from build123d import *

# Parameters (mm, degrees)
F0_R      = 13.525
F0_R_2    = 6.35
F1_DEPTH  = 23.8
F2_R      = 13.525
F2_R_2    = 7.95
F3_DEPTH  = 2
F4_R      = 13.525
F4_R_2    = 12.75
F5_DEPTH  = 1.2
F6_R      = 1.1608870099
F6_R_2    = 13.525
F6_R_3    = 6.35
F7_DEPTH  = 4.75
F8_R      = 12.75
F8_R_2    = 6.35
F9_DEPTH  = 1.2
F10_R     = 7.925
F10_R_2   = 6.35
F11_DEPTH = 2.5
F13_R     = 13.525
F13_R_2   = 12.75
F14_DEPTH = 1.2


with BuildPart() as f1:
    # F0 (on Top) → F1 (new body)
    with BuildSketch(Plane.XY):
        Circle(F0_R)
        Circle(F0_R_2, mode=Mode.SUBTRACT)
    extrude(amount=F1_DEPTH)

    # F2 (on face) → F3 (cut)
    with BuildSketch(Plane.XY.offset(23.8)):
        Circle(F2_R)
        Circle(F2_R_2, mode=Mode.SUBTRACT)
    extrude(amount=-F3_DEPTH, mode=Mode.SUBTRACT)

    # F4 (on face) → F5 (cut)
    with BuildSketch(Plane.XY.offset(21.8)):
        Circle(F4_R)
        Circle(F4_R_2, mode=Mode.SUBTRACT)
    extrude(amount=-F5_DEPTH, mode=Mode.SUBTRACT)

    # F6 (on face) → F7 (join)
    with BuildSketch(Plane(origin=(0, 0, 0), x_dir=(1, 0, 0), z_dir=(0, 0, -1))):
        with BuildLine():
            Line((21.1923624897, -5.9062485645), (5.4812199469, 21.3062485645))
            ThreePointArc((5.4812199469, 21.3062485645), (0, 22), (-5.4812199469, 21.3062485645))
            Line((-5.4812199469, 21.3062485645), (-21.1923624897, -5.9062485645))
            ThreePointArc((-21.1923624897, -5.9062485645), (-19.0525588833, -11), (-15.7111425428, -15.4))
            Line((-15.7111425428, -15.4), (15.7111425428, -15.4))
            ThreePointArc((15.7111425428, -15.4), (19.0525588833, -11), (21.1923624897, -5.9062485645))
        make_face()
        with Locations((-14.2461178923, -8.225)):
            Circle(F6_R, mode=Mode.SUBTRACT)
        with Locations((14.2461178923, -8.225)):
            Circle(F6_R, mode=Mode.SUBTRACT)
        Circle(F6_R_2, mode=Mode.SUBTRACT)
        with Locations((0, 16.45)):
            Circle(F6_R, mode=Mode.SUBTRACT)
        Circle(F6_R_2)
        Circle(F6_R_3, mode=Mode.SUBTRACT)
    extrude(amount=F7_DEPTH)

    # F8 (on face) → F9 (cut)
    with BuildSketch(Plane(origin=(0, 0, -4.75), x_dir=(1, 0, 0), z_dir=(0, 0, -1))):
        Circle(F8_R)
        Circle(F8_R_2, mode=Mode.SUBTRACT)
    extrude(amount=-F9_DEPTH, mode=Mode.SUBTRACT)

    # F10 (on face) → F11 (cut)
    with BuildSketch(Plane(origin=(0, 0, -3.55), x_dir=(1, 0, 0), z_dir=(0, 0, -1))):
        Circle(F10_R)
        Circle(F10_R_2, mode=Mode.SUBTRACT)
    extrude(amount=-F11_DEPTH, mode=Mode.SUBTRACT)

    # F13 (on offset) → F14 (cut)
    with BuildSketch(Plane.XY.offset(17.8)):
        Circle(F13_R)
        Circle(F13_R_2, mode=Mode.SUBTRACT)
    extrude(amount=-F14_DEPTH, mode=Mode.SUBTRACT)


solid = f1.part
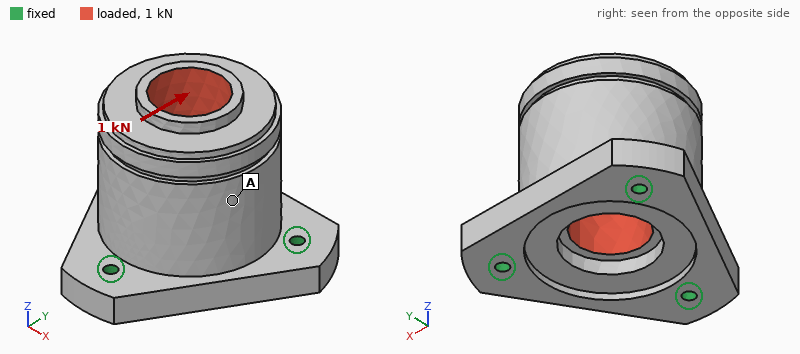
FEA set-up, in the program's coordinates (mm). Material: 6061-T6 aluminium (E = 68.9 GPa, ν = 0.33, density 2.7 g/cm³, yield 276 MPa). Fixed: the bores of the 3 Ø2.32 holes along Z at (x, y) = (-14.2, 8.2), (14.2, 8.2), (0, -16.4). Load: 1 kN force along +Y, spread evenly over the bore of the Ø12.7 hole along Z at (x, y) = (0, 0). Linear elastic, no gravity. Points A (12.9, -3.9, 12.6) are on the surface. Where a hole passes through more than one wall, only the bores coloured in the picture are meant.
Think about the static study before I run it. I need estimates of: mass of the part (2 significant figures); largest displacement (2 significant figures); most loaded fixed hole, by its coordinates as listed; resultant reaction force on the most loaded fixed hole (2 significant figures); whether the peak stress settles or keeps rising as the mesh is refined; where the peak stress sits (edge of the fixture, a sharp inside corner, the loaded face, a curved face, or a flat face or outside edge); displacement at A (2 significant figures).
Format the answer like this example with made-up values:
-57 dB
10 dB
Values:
37 g
11 µm
(0, -16.4)
730 N
keeps rising
edge of the fixture
6.2 µm
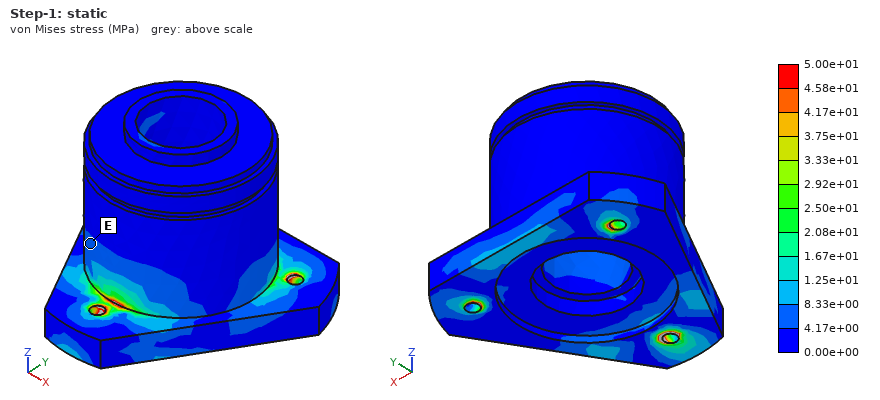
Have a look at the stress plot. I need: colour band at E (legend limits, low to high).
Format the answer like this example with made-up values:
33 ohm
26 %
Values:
4.17e+00 to 8.33e+00 MPa
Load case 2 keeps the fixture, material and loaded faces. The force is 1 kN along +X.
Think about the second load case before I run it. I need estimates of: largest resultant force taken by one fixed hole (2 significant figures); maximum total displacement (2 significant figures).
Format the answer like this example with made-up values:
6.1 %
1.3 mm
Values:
640 N
11 µm
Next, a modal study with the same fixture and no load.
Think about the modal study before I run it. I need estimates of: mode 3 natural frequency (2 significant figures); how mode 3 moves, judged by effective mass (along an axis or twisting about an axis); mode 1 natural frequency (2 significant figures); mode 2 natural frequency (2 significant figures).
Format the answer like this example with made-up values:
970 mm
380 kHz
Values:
17 kHz
along Z
11 kHz
11 kHz
